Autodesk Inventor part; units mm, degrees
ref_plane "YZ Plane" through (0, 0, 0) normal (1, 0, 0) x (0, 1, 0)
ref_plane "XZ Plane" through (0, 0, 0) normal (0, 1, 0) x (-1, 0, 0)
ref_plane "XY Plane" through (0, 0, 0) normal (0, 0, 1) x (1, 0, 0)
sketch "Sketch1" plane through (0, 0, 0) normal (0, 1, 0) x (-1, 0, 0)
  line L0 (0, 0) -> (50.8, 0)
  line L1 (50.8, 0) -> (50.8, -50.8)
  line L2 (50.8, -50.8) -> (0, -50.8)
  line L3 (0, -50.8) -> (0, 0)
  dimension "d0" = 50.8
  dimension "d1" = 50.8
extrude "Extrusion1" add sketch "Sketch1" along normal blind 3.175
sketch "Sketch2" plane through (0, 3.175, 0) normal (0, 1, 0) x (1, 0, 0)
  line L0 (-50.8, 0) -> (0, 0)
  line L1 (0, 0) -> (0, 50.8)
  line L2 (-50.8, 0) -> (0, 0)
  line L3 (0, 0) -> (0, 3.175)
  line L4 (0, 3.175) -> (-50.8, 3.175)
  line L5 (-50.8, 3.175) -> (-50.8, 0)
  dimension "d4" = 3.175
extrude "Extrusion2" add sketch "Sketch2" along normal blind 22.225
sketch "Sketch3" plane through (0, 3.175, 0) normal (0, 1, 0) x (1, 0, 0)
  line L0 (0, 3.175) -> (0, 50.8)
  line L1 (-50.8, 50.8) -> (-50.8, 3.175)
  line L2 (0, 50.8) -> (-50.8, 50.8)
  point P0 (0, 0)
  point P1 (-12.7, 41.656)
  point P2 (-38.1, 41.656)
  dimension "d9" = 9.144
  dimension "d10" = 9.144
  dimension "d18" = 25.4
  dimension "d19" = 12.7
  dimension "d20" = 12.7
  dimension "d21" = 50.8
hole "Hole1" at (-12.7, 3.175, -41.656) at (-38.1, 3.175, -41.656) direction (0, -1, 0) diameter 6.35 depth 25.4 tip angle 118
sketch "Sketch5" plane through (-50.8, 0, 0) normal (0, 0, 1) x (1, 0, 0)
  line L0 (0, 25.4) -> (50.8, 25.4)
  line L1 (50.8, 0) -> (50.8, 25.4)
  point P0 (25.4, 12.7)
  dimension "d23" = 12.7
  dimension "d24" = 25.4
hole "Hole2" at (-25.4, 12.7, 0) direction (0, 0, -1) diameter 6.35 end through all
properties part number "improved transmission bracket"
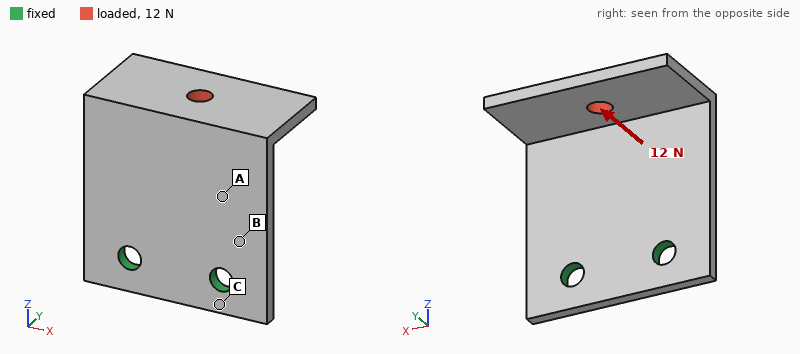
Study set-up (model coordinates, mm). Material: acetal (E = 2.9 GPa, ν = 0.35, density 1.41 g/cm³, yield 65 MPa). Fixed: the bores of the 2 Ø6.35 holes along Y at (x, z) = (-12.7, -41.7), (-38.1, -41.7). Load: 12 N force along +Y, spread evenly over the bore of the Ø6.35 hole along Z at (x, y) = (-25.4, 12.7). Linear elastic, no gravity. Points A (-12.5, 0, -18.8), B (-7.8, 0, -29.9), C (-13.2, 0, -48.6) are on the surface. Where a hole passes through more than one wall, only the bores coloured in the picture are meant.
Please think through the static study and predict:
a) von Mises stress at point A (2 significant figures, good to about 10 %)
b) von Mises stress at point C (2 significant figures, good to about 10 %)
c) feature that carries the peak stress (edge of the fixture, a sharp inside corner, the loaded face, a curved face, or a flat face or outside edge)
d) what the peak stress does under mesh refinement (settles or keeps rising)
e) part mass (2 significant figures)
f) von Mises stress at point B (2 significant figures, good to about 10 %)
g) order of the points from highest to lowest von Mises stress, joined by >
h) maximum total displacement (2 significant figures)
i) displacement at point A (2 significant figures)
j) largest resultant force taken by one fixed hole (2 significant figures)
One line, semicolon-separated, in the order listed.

2.2 MPa; 0.86 MPa; edge of the fixture; keeps rising; 16 g; 3.7 MPa; B > A > C; 0.78 mm; 0.22 mm; 6.0 N
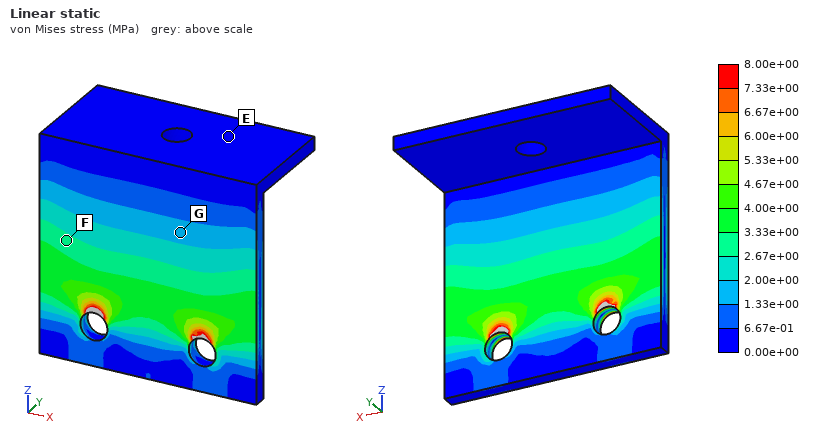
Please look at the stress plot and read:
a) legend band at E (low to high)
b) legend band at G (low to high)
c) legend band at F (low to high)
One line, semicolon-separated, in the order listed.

0.00e+00 to 6.67e-01 MPa; 1.33e+00 to 2.00e+00 MPa; 2.67e+00 to 3.33e+00 MPa
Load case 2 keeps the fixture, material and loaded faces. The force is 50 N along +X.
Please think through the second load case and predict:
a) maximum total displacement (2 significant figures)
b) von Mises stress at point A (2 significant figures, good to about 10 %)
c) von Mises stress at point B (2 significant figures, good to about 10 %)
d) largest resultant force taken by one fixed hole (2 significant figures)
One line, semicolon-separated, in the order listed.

0.79 mm; 3.4 MPa; 3.8 MPa; 72 N
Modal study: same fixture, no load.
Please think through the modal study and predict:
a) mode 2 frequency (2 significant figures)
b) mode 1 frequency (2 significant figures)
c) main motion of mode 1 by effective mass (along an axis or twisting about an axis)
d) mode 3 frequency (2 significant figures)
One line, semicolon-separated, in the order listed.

480 Hz; 250 Hz; along Y; 870 Hz
